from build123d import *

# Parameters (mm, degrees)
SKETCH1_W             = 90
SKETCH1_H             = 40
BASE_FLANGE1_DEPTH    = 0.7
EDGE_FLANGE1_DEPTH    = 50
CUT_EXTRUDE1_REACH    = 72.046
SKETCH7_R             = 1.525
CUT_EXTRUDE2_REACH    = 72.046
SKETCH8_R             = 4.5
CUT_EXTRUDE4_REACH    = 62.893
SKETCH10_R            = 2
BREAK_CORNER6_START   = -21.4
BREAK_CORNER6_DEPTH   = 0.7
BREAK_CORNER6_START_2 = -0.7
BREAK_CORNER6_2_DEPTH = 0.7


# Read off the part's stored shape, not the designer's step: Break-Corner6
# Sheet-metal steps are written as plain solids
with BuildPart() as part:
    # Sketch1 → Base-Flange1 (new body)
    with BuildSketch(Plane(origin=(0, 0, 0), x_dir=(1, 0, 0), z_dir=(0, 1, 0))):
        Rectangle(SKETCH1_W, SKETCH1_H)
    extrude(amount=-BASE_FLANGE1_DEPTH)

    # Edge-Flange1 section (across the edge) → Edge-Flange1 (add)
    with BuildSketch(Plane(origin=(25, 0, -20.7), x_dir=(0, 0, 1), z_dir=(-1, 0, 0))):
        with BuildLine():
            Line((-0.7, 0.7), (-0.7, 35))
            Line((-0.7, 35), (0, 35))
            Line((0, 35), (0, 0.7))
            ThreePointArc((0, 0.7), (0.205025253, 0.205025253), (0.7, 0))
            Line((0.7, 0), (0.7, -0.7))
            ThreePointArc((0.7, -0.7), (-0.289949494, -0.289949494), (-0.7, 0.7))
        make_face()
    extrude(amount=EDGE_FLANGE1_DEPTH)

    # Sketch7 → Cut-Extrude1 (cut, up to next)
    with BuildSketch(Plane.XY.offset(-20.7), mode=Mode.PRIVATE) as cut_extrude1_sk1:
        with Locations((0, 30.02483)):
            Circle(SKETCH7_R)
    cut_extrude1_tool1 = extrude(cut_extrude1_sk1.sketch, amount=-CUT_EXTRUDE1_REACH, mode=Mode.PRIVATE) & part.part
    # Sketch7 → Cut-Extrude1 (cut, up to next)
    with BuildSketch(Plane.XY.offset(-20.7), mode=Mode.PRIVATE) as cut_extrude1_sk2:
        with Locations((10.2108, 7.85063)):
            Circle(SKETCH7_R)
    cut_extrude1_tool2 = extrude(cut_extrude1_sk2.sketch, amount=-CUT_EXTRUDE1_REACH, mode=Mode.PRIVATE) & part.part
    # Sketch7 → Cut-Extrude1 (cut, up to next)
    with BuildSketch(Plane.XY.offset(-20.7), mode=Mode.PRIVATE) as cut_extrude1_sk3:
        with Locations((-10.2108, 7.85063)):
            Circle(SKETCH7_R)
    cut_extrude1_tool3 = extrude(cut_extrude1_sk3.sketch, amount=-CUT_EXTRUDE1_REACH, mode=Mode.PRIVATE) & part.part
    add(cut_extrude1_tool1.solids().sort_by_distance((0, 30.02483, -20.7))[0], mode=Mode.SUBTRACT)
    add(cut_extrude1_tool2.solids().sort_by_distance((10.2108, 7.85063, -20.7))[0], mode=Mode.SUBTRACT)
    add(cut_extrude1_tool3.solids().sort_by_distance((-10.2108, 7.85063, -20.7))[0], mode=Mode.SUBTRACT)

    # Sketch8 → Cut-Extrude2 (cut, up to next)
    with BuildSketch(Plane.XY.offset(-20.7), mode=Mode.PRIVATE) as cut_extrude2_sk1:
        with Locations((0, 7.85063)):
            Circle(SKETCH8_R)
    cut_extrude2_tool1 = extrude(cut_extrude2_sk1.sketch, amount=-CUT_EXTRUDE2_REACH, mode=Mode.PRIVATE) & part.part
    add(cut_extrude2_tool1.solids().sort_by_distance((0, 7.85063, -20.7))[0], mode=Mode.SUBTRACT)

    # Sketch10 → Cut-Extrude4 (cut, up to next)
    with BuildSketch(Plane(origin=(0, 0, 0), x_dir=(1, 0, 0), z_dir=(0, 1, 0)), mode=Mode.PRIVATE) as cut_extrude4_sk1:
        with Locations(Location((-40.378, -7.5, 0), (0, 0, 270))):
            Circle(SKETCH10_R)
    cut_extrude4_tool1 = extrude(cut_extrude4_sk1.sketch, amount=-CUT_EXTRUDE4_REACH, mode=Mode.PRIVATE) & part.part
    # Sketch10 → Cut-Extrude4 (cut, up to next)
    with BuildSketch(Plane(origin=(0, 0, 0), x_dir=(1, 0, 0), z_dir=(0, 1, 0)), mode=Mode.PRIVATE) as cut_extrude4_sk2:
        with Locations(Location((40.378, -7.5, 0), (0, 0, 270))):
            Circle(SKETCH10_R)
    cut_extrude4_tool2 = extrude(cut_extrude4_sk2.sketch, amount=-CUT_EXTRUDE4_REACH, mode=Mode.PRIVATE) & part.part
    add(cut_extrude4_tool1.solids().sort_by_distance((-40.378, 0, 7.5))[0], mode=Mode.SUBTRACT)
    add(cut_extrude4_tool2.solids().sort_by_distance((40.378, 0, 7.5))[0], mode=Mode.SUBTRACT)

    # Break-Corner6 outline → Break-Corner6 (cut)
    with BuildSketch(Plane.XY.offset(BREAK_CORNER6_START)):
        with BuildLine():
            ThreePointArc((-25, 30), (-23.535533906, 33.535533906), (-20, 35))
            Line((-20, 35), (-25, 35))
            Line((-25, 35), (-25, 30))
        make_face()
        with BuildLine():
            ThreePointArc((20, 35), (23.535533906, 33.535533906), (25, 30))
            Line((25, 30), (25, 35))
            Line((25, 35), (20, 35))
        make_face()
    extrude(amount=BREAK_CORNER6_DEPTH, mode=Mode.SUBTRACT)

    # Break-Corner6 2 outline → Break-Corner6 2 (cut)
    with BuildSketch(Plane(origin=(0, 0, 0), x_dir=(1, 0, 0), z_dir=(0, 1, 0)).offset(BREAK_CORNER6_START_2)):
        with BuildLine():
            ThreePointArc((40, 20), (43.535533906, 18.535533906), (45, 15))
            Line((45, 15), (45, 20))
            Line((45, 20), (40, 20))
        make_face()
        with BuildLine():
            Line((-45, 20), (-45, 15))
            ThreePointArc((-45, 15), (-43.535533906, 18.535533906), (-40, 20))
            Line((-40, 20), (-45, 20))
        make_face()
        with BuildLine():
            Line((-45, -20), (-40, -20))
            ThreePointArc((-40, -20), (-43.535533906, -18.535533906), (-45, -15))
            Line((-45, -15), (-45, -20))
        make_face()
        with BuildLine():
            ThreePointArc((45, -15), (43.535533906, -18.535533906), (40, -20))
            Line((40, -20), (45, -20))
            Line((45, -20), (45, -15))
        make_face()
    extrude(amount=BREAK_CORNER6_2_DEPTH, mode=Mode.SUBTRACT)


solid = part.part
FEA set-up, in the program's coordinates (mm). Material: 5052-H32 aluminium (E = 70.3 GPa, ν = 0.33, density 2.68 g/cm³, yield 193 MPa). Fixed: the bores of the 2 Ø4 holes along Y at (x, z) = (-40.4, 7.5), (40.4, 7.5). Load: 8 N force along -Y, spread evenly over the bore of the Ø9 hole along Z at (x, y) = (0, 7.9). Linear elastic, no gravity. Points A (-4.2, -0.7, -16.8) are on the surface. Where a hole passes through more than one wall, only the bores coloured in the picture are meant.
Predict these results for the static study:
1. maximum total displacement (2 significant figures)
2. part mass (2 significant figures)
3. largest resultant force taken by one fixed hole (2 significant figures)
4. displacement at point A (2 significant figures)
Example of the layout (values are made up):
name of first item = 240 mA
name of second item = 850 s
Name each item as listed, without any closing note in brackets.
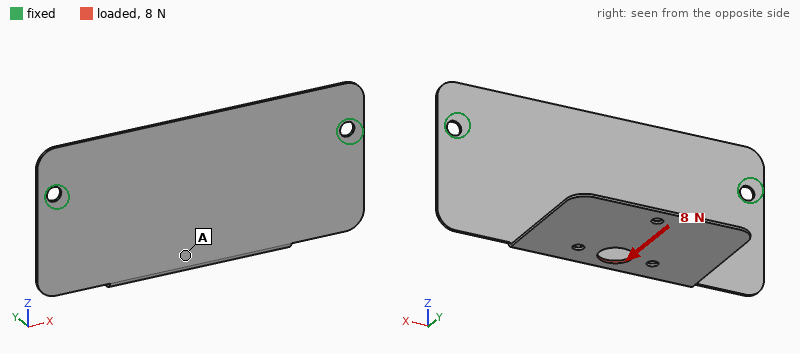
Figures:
maximum total displacement = 1.2 mm
part mass = 9.9 g
largest resultant force taken by one fixed hole = 4.0 N
displacement at point A = 0.61 mm
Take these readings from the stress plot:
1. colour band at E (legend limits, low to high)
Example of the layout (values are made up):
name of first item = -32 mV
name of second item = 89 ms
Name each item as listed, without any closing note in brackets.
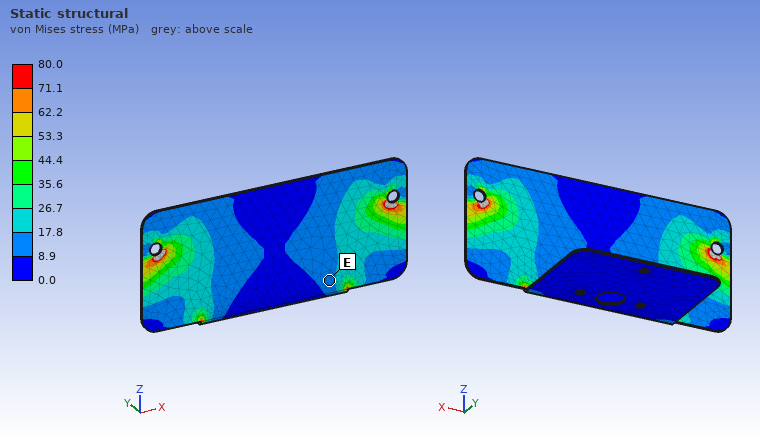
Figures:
colour band at E = 8.9 to 17.8 MPa
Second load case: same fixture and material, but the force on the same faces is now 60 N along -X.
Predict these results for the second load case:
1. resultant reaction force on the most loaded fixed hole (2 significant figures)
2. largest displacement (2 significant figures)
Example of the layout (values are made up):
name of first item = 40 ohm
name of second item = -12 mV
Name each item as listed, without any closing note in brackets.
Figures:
resultant reaction force on the most loaded fixed hole = 37 N
largest displacement = 1.1 mm
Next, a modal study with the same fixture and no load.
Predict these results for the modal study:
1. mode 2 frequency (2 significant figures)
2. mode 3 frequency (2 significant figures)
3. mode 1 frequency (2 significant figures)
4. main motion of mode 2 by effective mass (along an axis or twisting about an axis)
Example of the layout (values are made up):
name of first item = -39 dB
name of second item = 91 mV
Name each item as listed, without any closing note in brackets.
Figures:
mode 2 frequency = 400 Hz
mode 3 frequency = 440 Hz
mode 1 frequency = 200 Hz
main motion of mode 2 by effective mass = along Y
